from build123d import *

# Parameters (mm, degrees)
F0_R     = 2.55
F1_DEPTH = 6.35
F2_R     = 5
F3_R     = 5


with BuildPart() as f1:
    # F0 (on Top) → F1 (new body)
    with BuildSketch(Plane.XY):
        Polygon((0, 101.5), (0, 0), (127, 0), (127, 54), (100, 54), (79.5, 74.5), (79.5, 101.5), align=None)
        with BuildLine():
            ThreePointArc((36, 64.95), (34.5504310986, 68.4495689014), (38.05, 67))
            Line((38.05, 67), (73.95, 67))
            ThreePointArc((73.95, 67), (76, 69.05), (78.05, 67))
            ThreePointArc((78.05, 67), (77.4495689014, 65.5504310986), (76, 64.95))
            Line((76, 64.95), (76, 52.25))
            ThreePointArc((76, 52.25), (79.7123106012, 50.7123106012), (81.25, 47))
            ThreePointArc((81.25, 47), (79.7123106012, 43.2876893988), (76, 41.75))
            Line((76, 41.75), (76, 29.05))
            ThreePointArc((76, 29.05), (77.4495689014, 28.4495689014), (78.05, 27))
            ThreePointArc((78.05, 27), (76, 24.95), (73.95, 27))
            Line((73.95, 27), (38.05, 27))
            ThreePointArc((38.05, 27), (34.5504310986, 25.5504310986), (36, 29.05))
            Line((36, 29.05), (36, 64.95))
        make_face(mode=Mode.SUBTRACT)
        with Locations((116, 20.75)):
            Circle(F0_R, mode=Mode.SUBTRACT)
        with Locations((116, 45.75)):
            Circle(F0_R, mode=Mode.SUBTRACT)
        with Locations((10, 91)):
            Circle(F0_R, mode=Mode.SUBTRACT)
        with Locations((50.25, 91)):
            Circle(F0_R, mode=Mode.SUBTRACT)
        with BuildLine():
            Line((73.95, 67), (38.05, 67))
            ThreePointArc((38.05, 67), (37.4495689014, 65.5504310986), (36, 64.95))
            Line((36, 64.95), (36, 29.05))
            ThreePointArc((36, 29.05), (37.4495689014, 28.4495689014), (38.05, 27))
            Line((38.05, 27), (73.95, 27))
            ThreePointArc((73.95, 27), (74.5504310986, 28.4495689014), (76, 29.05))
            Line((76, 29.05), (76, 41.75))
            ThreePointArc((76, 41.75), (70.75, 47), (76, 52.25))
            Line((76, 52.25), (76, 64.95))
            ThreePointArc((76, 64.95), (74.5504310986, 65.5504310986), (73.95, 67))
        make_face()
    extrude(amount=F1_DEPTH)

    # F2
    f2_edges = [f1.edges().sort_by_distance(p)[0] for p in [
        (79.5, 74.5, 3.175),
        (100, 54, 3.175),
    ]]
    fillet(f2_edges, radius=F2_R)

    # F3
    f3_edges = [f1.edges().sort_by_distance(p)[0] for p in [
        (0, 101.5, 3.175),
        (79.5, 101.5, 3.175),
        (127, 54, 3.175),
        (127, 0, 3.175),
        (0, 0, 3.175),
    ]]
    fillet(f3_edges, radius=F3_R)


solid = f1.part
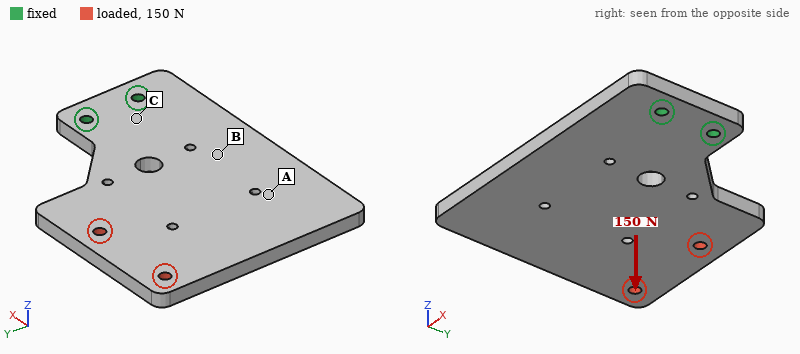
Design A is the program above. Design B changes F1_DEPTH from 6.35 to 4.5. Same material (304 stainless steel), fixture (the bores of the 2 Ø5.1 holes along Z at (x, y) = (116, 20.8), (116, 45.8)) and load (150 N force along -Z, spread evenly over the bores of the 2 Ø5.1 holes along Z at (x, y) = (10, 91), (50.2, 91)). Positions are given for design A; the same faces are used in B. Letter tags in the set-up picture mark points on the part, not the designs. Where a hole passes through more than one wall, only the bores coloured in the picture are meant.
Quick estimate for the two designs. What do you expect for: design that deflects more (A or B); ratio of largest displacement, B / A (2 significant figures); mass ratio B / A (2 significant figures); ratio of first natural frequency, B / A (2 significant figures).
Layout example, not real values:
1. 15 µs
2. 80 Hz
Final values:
1. B
2. 2.7
3. 0.71
4. 0.72
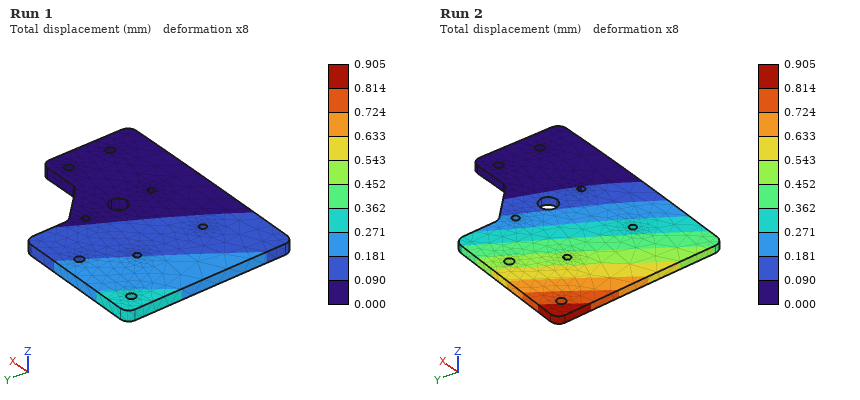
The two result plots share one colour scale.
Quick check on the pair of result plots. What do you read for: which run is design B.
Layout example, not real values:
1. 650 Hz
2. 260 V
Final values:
1. Run 2
